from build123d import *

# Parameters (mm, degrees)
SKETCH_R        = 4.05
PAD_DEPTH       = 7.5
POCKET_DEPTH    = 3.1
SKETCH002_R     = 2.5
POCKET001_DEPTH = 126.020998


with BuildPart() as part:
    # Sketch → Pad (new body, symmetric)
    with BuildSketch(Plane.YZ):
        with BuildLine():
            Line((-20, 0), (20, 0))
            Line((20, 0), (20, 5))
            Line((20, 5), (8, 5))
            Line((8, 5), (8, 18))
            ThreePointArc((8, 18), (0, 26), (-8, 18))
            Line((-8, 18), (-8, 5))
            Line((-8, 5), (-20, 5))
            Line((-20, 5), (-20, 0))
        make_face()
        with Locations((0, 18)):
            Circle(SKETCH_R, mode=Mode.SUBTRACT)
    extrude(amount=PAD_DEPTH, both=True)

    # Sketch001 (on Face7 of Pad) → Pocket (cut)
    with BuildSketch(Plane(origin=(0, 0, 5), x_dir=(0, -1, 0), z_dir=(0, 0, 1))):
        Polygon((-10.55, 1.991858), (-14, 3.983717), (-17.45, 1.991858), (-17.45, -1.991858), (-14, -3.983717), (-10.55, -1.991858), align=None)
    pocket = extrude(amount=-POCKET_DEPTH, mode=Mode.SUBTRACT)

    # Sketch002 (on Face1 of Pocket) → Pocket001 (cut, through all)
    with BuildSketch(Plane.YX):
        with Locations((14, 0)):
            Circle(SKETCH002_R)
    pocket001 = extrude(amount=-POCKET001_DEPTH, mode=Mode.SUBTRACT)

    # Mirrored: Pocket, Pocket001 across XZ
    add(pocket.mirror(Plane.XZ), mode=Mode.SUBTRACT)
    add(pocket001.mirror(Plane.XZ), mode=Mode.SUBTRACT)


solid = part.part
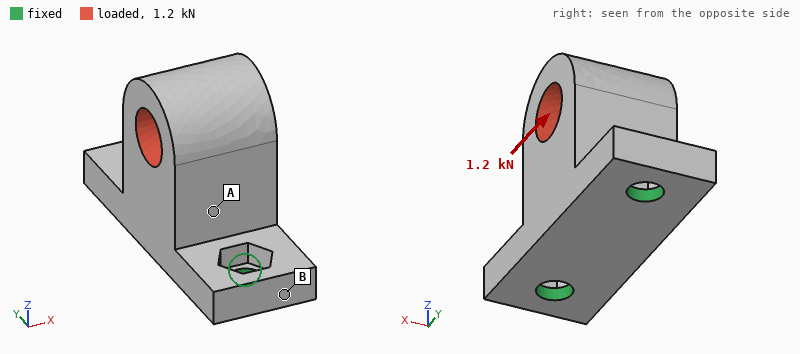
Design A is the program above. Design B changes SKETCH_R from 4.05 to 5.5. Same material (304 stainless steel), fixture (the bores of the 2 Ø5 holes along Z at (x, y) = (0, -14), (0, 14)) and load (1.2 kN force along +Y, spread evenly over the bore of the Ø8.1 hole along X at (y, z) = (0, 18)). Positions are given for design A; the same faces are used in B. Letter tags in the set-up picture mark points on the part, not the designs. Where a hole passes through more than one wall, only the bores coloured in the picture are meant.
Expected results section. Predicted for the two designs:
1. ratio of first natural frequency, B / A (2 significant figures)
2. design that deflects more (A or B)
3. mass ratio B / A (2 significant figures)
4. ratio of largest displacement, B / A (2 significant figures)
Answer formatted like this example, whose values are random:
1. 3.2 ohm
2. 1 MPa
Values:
1. 1.1
2. B
3. 0.90
4. 1.4
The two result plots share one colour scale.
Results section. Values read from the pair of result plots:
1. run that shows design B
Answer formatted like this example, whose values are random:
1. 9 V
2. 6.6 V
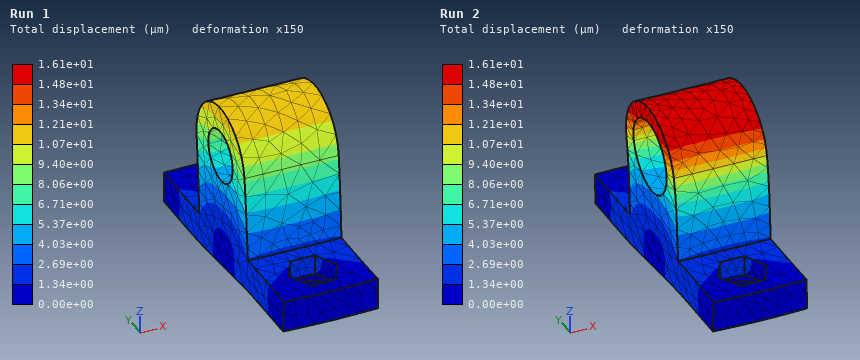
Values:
1. Run 2
